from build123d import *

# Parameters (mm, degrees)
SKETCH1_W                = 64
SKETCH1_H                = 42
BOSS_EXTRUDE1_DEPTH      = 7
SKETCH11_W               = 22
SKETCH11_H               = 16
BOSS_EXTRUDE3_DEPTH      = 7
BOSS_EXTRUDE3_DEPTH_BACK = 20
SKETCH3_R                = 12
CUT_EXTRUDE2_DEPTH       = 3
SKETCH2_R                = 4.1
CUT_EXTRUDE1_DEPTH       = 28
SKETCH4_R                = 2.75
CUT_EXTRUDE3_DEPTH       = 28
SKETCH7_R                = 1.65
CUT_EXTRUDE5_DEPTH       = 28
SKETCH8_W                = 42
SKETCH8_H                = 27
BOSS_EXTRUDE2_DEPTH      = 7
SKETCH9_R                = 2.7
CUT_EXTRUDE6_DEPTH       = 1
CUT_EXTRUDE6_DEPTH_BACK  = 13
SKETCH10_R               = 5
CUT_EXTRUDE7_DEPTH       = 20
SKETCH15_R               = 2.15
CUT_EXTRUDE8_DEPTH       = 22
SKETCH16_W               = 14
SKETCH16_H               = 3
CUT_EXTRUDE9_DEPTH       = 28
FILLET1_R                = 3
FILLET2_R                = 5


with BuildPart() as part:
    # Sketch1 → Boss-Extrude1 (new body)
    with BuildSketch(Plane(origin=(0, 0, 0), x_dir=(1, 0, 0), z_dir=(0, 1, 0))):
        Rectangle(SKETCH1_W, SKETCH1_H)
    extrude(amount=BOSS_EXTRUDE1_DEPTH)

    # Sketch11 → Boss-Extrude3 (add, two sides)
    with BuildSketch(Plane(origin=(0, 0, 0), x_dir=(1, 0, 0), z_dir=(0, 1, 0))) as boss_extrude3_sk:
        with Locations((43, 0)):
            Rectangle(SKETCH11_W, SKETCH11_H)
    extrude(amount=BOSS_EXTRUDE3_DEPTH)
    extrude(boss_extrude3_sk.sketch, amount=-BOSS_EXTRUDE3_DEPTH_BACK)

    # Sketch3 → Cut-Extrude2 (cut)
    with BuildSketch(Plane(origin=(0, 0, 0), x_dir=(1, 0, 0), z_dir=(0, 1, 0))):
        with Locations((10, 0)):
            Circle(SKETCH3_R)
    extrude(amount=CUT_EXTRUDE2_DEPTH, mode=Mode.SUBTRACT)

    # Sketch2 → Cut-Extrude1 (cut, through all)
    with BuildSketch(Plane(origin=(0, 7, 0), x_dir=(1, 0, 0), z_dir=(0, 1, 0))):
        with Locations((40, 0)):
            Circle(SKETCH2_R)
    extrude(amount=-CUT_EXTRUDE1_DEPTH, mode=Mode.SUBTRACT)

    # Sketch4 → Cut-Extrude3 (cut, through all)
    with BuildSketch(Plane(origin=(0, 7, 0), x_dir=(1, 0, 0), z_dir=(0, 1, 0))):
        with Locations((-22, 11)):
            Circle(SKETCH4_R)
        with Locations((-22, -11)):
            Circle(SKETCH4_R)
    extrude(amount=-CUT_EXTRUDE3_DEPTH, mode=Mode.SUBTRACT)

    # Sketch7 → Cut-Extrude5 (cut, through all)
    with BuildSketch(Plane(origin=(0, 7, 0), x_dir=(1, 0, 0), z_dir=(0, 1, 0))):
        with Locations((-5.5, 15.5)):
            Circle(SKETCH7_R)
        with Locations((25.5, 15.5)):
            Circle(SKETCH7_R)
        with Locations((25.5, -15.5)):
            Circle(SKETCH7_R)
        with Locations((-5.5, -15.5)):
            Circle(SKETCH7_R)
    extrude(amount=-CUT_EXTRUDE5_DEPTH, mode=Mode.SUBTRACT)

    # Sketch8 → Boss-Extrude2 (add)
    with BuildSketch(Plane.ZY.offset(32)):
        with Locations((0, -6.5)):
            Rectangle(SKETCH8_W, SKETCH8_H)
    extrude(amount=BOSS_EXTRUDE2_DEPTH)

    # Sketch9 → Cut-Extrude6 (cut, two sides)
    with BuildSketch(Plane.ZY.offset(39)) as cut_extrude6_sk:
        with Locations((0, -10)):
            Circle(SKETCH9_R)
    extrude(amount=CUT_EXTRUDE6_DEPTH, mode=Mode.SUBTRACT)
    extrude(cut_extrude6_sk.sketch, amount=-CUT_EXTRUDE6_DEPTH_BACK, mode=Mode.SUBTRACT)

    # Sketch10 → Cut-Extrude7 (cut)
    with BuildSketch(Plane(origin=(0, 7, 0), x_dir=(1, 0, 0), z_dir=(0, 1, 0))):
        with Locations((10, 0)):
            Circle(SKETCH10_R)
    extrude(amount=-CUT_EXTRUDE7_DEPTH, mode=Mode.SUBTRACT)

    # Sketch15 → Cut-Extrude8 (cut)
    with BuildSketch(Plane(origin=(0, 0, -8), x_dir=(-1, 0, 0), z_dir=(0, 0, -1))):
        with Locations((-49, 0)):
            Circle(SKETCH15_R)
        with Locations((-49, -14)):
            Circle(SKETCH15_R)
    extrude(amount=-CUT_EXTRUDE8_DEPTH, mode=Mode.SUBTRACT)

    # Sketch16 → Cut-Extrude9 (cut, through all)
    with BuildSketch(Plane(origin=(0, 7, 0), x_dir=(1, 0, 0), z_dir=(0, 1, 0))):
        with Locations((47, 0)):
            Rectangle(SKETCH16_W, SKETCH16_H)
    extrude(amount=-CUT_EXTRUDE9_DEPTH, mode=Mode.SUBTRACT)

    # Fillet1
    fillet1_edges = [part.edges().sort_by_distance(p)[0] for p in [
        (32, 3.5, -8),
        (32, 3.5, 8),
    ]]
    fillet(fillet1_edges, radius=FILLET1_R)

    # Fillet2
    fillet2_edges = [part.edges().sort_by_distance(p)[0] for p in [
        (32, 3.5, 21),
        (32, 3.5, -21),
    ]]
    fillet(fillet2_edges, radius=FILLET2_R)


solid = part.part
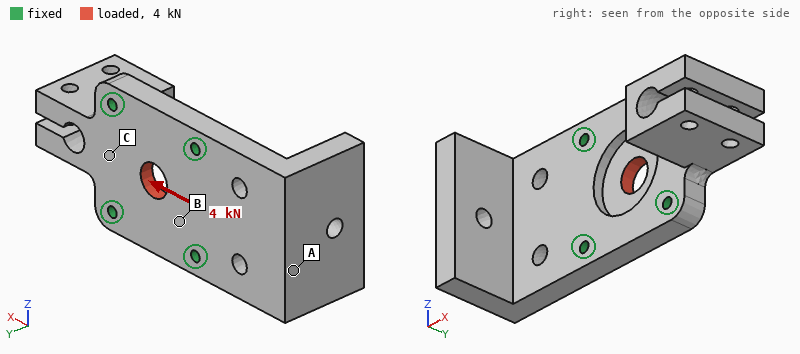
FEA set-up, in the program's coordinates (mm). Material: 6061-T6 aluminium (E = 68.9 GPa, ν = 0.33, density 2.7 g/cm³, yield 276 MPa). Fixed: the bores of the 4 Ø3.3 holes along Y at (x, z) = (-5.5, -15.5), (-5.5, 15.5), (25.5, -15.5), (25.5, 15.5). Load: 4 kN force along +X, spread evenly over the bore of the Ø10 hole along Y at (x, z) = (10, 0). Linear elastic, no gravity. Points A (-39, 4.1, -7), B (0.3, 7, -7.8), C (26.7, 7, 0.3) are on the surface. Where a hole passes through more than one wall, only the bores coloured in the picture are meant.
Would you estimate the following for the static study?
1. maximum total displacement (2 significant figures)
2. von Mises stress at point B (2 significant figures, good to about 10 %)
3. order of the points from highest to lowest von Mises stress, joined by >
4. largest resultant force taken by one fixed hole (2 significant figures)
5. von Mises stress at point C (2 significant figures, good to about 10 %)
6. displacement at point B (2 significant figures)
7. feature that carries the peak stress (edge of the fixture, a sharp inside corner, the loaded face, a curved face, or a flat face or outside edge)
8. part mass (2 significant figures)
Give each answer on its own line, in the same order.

7.3 µm
18 MPa
B > C > A
1.1 kN
9.8 MPa
3.0 µm
the loaded face
84 g
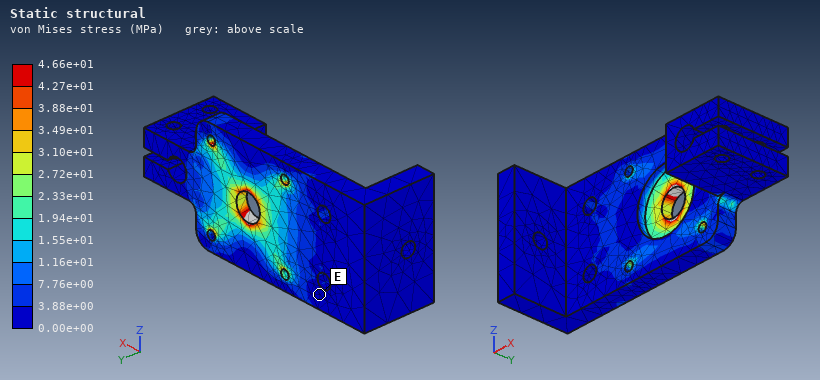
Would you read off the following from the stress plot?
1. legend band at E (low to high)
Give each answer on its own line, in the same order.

0.00e+00 to 3.88e+00 MPa
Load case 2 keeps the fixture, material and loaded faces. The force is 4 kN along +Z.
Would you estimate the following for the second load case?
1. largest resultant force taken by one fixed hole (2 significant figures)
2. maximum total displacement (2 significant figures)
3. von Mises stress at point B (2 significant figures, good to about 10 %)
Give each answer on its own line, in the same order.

1.1 kN
7.9 µm
20 MPa
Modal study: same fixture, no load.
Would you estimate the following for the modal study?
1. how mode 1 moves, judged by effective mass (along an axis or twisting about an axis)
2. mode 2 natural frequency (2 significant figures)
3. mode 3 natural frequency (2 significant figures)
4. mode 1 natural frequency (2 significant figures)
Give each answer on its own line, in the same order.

along Y
3000 Hz
4600 Hz
2300 Hz
